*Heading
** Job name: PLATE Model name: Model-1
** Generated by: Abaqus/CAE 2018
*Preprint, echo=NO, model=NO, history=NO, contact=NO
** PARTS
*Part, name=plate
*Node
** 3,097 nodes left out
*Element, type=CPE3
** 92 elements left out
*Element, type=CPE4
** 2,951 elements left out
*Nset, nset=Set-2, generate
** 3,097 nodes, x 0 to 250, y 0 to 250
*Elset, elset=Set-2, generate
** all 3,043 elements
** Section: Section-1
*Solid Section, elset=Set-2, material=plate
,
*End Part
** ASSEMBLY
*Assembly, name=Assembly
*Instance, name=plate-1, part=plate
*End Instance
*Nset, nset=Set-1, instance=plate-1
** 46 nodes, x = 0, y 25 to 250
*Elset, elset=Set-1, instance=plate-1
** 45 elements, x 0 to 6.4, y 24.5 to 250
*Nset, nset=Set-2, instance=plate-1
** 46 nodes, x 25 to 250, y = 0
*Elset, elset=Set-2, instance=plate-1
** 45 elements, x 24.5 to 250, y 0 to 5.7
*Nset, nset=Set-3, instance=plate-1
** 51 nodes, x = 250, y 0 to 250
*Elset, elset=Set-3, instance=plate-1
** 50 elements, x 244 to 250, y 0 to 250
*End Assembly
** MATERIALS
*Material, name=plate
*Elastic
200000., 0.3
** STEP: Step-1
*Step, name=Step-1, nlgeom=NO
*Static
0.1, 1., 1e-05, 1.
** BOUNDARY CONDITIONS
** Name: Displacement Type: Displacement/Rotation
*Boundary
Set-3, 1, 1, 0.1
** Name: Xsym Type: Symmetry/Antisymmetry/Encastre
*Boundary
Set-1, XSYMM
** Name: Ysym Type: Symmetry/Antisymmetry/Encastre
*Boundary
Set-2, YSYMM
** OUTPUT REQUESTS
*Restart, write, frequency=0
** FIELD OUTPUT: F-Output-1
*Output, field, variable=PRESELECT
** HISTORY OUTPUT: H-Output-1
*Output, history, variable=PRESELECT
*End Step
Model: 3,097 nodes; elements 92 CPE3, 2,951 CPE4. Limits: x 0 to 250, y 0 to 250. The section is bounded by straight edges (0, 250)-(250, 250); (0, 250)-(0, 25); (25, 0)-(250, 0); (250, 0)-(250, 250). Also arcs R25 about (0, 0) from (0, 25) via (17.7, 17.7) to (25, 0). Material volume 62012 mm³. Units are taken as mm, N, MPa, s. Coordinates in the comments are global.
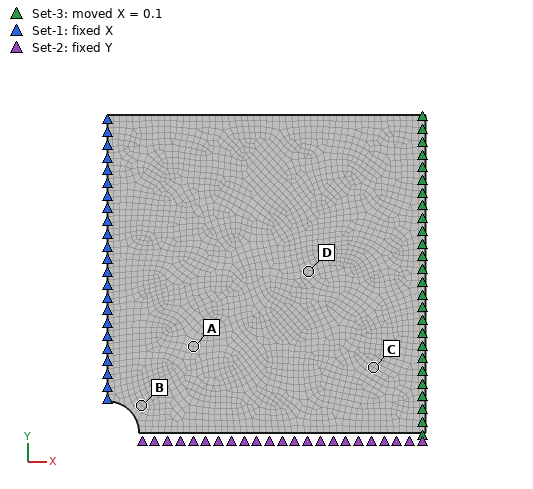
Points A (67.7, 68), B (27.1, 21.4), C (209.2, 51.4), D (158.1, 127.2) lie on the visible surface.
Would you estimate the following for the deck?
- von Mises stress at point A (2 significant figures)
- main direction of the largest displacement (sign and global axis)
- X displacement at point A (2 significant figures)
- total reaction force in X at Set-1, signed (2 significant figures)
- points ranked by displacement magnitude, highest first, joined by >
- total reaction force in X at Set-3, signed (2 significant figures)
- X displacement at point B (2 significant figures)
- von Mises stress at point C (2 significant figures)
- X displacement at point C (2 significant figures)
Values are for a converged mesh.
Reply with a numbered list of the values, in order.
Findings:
1. 86 MPa
2. +X
3. 0.029 mm
4. -21000 N
5. C > D > A > B
6. 21000 N
7. 0.021 mm
8. 73 MPa
9. 0.085 mm
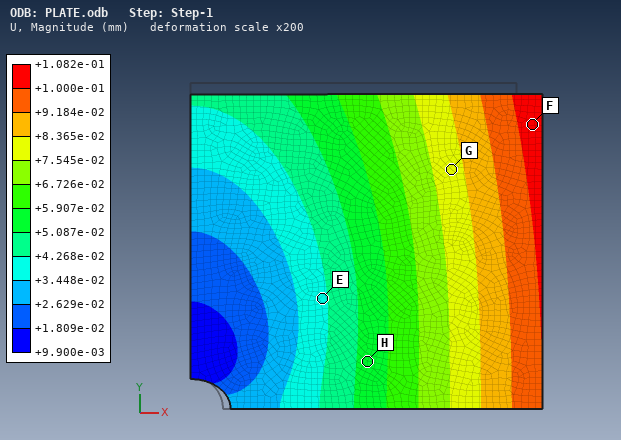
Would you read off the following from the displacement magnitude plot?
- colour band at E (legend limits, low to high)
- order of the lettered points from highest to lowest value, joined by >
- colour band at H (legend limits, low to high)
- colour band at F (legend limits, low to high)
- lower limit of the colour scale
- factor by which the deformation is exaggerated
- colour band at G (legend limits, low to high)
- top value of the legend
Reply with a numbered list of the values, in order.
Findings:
1. +3.448e-02 to +4.268e-02 mm
2. F > G > H > E
3. +5.087e-02 to +5.907e-02 mm
4. +1.000e-01 to +1.082e-01 mm
5. +9.900e-03 mm
6. 200
7. +7.545e-02 to +8.365e-02 mm
8. +1.082e-01 mm
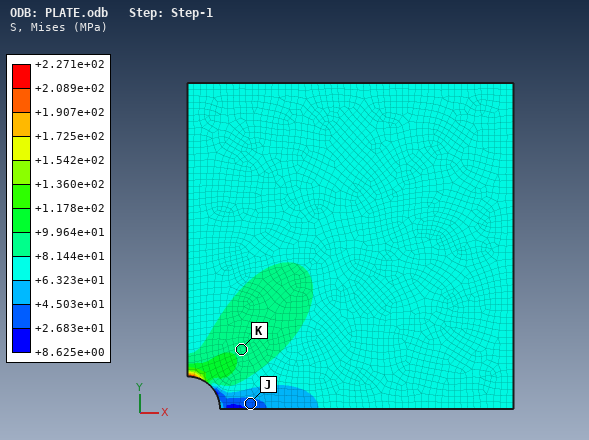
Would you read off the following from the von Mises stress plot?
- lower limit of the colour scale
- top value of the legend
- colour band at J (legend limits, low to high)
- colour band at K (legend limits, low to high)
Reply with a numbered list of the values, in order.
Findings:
1. +8.625e+00 MPa
2. +2.271e+02 MPa
3. +2.683e+01 to +4.503e+01 MPa
4. +8.144e+01 to +9.964e+01 MPa
